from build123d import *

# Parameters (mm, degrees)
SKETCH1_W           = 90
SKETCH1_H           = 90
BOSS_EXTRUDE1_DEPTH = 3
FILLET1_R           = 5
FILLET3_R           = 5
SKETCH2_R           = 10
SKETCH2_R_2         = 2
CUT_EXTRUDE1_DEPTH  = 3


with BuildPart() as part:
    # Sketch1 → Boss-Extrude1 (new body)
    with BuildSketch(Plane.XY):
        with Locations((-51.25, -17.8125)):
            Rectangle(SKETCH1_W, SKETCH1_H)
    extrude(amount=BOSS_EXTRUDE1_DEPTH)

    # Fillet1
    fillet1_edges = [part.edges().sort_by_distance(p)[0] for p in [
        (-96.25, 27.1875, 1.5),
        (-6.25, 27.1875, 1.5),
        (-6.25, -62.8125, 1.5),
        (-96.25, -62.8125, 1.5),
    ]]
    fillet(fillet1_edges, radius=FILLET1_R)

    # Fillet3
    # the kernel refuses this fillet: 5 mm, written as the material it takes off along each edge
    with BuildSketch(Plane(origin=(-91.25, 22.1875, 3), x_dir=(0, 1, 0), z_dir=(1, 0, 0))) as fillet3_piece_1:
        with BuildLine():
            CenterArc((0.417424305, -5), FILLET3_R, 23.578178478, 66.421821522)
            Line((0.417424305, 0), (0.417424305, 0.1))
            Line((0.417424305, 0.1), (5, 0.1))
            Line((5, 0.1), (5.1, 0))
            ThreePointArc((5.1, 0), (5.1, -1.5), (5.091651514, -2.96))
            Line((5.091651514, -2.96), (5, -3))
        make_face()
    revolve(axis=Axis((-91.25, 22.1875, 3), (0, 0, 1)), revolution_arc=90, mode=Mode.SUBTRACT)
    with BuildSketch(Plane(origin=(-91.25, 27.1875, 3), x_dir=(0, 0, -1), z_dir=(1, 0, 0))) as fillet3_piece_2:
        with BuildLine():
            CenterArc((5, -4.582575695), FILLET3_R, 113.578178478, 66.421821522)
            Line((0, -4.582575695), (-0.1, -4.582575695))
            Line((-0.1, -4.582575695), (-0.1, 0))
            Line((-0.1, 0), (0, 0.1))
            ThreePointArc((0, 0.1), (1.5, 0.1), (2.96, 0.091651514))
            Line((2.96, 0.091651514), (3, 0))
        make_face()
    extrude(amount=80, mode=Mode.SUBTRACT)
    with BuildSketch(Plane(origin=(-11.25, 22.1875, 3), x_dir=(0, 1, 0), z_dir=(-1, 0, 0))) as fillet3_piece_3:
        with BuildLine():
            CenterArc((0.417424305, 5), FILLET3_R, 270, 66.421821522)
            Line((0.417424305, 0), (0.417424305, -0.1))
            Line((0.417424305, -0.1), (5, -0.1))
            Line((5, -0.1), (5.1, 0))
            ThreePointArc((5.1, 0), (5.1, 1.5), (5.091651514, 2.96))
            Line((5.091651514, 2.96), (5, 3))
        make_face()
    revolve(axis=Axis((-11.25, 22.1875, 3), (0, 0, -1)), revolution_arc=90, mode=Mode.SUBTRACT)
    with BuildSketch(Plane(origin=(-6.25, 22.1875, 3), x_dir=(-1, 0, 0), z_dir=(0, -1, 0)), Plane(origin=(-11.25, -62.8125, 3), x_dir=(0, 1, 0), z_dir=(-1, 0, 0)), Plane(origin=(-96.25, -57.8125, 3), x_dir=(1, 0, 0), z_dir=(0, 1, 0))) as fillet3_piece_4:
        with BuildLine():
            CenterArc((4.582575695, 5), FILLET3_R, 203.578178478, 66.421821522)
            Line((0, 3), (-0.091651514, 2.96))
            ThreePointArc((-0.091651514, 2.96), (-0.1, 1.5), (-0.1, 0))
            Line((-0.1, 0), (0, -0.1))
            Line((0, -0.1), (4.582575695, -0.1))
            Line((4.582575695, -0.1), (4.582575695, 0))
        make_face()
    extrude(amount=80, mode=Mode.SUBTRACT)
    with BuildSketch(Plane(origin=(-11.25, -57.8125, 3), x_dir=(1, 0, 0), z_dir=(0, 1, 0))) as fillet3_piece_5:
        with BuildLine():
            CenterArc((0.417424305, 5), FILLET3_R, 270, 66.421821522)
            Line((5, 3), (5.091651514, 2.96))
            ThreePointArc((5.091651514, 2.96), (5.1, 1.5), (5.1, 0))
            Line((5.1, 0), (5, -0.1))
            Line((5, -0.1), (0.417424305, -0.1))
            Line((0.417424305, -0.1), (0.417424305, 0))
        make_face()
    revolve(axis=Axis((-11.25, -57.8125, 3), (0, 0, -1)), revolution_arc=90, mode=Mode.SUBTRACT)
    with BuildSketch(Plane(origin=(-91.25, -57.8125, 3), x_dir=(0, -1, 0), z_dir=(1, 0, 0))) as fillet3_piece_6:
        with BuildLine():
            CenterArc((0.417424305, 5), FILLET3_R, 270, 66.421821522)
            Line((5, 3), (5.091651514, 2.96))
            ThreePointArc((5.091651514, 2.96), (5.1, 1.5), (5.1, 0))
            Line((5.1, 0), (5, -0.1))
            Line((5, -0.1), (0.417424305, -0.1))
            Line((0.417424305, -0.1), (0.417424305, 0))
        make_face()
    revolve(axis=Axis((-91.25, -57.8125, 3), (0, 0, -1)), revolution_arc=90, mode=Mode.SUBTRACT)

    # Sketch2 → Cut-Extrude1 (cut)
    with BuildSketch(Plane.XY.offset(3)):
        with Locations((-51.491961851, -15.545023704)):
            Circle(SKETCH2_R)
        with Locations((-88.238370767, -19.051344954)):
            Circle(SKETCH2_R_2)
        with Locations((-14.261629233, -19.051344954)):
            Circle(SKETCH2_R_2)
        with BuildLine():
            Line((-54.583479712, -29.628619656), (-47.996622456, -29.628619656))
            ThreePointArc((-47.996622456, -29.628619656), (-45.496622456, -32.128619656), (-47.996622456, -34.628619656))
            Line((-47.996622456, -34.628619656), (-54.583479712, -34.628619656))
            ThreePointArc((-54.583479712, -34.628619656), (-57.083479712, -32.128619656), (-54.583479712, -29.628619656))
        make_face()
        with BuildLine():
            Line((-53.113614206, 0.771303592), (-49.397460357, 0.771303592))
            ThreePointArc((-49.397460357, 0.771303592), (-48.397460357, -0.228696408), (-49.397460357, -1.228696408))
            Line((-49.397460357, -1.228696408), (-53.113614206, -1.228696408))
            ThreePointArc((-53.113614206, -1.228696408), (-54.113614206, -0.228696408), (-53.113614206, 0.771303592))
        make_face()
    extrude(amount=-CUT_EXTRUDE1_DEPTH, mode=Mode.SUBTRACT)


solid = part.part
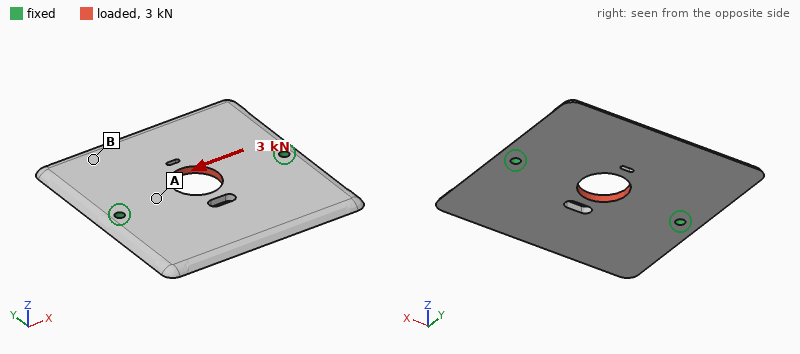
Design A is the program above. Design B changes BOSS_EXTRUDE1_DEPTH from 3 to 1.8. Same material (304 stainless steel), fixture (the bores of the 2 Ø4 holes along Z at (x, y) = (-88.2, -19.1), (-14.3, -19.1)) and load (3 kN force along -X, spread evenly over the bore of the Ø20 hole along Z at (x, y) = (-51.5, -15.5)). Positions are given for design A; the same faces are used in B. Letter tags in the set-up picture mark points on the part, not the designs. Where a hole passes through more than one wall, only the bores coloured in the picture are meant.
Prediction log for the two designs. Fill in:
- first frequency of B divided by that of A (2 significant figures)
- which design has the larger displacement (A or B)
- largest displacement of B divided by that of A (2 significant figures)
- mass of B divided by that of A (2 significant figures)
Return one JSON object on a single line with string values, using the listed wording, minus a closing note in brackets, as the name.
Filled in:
{"first frequency of B divided by that of A": "0.62", "which design has the larger displacement": "B", "largest displacement of B divided by that of A": "1.6", "mass of B divided by that of A": "0.62"}
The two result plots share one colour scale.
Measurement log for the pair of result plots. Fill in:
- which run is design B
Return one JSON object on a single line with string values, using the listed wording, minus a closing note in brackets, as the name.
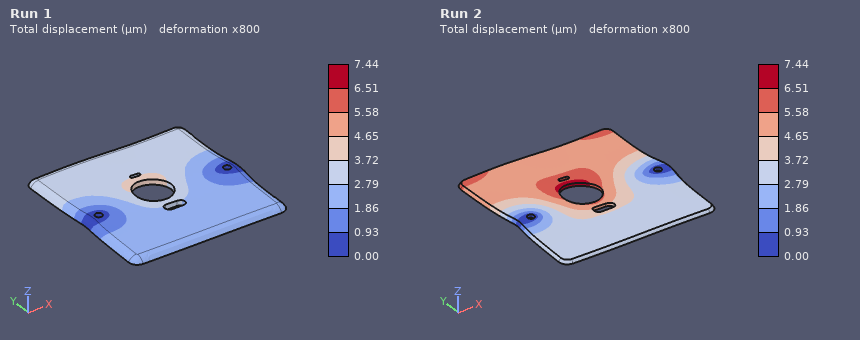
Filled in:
{"which run is design B": "Run 2"}
